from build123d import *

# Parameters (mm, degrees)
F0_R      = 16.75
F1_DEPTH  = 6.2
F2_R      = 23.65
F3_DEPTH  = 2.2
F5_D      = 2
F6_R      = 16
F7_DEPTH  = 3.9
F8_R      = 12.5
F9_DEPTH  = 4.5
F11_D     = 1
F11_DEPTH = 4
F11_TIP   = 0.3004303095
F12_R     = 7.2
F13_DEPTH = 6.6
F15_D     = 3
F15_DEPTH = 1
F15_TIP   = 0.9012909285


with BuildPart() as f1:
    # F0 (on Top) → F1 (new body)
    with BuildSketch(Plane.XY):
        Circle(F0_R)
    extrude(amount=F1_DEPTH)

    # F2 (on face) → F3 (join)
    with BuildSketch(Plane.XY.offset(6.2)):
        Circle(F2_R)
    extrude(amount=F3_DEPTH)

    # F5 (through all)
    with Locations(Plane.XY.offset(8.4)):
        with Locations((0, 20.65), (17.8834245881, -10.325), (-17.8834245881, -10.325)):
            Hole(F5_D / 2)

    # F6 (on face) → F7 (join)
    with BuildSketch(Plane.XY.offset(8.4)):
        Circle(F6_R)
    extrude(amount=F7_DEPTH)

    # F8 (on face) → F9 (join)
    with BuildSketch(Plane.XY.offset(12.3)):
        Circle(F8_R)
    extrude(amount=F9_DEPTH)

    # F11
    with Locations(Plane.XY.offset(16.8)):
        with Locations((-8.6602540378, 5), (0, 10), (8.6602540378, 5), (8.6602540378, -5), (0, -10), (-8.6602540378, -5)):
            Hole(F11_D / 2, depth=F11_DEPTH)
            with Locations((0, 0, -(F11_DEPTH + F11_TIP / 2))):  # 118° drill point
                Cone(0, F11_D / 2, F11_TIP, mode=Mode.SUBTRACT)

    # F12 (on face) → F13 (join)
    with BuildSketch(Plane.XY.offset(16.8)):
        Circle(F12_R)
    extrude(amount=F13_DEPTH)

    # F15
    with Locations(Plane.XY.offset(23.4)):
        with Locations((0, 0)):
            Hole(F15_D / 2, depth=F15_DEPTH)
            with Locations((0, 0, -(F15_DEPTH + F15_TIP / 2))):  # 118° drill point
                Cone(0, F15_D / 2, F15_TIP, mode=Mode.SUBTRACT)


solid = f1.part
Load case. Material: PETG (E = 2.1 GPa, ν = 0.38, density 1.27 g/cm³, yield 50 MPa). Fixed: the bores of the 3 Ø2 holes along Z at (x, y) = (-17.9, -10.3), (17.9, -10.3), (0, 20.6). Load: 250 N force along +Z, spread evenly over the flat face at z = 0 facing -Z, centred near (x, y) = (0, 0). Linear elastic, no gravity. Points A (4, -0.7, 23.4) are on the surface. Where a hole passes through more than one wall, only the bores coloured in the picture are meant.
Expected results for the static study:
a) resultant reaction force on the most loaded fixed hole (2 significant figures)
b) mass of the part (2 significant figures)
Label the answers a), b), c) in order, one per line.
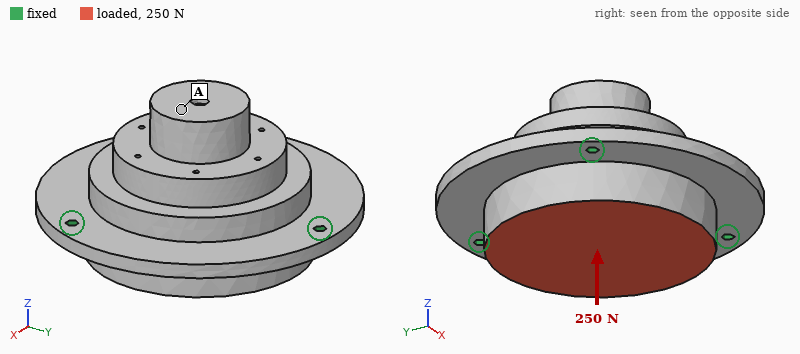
a) 85 N
b) 20 g
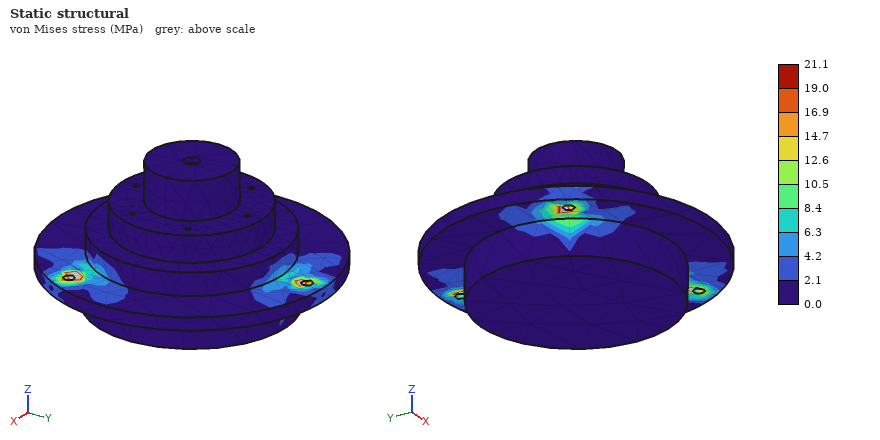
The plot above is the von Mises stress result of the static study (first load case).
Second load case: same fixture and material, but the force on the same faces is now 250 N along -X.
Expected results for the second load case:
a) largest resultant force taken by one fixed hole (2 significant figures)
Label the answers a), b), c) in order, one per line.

a) 110 N
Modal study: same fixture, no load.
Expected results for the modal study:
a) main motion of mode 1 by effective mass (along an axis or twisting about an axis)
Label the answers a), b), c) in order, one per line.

a) along Z
